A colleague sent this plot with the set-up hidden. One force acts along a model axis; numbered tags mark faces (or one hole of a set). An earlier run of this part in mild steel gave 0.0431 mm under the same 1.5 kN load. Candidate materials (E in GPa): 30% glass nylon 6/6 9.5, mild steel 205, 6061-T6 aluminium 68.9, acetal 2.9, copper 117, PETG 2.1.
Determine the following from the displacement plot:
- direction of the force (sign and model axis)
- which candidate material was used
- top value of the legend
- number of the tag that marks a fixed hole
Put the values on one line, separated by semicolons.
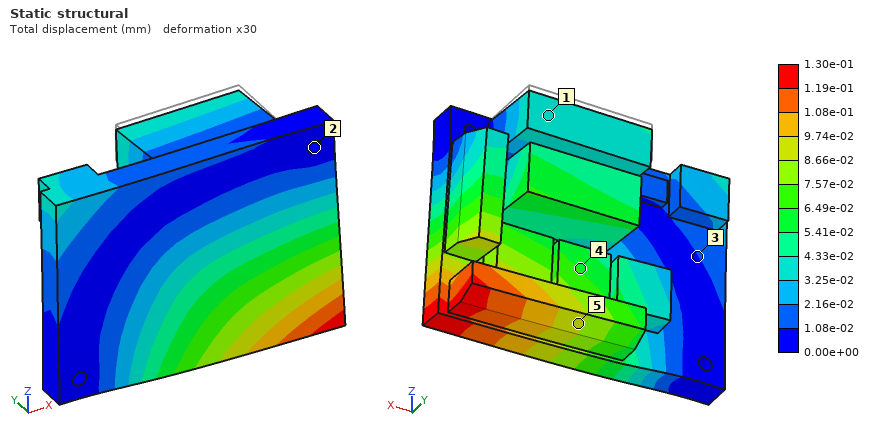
-Y; 6061-T6 aluminium; 1.30e-01 mm; 2
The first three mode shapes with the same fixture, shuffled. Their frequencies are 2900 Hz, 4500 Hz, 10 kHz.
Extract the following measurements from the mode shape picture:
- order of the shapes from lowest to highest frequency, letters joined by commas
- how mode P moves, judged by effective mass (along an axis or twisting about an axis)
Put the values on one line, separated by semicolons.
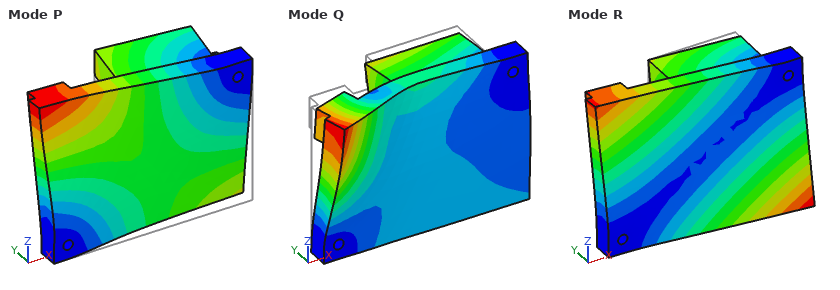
R, P, Q; along Y
